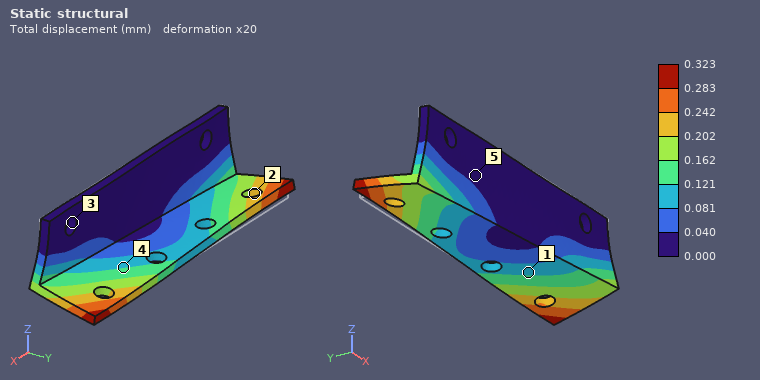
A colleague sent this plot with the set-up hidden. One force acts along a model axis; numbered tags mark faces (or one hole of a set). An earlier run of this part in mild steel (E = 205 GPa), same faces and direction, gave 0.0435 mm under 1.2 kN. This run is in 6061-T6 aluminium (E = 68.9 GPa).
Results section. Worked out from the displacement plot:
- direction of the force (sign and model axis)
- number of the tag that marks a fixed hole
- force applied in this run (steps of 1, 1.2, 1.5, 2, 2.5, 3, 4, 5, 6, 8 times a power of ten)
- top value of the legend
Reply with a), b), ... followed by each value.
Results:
a) +X
b) 3
c) 3 kN
d) 0.323 mm
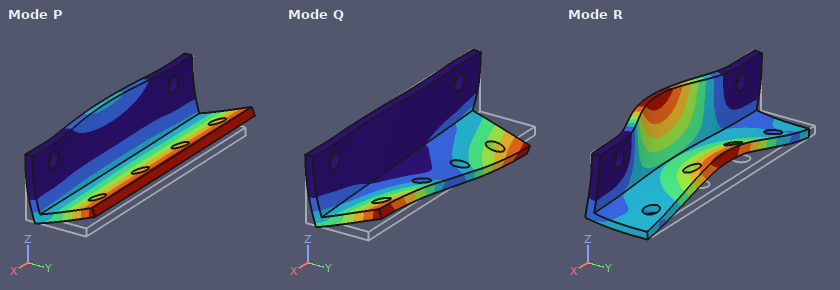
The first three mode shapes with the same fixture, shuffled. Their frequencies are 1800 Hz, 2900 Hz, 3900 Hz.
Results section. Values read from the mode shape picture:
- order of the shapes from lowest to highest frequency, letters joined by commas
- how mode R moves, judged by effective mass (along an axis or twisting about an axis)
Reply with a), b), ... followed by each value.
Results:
a) P, Q, R
b) along Y
